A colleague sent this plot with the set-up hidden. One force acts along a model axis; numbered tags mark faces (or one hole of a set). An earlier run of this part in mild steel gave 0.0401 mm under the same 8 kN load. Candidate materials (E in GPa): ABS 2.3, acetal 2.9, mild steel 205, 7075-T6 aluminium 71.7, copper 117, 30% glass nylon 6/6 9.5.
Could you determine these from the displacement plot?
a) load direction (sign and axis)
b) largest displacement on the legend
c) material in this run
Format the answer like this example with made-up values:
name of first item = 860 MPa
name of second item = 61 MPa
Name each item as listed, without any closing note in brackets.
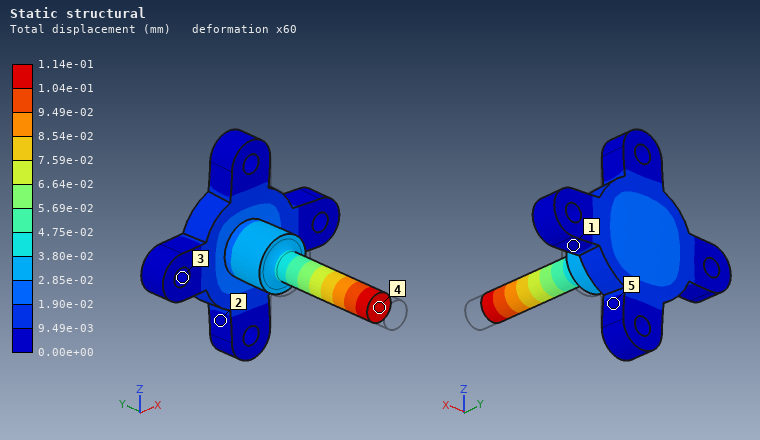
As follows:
load direction = +Y
largest displacement on the legend = 1.14e-01 mm
material in this run = 7075-T6 aluminium
